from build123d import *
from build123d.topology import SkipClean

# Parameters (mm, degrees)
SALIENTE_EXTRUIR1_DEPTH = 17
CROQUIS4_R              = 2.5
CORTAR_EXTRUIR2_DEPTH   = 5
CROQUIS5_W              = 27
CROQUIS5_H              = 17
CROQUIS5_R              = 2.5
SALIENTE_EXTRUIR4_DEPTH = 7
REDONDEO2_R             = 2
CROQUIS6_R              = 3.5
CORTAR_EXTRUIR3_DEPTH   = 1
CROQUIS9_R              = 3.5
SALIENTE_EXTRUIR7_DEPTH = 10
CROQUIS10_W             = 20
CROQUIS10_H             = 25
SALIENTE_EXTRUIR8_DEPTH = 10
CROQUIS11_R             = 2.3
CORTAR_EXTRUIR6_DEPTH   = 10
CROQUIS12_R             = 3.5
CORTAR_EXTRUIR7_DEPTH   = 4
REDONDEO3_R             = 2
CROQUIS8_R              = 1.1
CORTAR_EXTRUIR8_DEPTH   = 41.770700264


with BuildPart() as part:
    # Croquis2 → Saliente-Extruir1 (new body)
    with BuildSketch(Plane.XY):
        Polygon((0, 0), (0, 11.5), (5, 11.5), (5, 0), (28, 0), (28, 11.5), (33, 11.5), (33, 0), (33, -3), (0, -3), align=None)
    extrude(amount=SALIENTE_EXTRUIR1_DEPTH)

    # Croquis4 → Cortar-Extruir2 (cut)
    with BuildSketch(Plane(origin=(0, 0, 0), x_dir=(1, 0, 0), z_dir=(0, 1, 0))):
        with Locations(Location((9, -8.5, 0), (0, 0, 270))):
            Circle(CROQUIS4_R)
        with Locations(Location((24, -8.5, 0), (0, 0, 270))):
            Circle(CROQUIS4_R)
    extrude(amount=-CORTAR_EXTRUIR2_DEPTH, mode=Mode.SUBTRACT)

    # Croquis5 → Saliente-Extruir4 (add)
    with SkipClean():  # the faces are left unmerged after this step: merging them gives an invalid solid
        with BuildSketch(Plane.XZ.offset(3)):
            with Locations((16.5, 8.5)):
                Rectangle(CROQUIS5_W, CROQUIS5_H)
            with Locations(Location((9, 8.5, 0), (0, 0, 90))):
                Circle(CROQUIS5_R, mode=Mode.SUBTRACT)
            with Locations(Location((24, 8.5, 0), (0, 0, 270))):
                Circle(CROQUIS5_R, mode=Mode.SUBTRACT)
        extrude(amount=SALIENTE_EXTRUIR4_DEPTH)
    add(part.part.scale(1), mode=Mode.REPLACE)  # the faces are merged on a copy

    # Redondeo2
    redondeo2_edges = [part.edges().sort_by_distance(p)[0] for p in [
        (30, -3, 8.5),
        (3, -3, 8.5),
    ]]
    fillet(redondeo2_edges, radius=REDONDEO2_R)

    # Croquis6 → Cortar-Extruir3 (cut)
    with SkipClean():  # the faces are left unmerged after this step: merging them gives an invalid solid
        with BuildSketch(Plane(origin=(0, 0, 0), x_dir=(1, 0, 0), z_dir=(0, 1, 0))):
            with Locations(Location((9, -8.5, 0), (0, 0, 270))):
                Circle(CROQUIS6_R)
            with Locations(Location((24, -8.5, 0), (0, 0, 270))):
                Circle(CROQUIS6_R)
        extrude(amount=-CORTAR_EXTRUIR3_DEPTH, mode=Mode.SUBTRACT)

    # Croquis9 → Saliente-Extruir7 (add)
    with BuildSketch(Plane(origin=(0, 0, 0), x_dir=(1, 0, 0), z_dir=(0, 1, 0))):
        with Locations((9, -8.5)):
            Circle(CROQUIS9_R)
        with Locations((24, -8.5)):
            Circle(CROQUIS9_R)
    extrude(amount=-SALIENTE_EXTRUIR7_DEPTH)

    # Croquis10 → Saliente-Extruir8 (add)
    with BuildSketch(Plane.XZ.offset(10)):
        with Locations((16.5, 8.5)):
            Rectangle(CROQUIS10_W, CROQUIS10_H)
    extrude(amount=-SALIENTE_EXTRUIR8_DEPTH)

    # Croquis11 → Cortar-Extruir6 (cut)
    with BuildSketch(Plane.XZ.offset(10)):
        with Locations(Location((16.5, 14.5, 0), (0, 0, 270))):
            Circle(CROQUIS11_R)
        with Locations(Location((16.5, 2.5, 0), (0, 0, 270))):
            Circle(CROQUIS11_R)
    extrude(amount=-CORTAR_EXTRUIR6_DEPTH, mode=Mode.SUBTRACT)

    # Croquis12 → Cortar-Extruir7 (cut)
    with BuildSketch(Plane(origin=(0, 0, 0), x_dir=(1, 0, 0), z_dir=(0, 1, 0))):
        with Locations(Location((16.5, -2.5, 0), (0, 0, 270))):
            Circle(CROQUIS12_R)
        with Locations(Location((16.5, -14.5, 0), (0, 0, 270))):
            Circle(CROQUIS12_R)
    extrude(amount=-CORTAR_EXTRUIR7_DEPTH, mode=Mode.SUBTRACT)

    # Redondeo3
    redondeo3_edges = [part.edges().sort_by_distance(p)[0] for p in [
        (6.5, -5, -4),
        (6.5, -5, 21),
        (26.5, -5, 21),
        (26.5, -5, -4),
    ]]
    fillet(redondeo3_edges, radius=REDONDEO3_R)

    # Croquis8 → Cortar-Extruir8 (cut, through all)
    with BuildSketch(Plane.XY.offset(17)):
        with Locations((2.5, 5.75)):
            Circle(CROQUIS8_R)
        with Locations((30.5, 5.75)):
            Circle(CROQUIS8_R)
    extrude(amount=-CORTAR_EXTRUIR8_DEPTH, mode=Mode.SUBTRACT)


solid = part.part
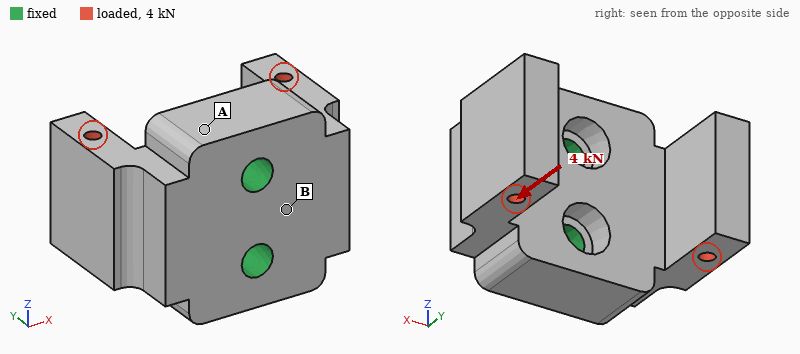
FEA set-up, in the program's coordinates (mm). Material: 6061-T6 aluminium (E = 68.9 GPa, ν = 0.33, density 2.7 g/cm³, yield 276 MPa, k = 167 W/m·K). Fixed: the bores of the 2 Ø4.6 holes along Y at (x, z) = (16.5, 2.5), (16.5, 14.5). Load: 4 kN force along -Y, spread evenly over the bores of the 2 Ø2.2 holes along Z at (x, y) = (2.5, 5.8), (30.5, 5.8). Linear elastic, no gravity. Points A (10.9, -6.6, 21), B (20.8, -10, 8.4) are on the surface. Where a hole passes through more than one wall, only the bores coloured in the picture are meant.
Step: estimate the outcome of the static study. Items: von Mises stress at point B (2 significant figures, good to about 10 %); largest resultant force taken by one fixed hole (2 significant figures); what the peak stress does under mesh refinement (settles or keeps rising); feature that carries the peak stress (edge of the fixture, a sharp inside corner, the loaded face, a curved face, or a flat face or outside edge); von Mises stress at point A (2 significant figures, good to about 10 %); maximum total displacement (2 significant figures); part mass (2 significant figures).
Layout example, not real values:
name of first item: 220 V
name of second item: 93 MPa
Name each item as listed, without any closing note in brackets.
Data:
von Mises stress at point B: 49 MPa
largest resultant force taken by one fixed hole: 2.0 kN
what the peak stress does under mesh refinement: keeps rising
feature that carries the peak stress: edge of the fixture
von Mises stress at point A: 20 MPa
maximum total displacement: 59 µm
part mass: 21 g
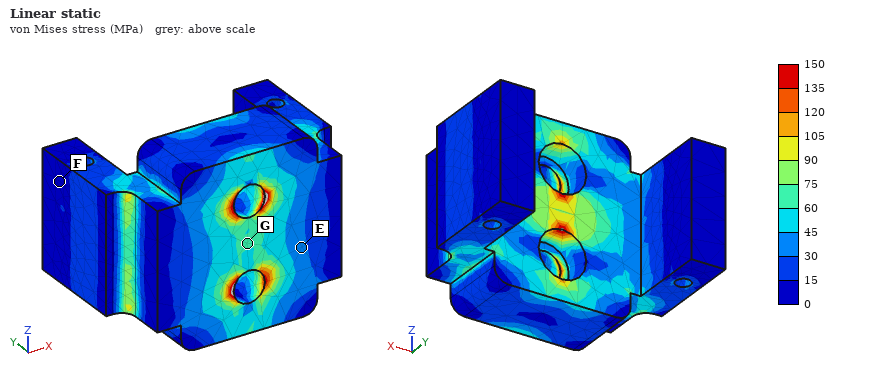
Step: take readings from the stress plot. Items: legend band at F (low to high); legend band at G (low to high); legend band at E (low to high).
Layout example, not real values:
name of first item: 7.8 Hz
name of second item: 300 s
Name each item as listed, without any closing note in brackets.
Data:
legend band at F: 0 to 15 MPa
legend band at G: 60 to 75 MPa
legend band at E: 30 to 45 MPa
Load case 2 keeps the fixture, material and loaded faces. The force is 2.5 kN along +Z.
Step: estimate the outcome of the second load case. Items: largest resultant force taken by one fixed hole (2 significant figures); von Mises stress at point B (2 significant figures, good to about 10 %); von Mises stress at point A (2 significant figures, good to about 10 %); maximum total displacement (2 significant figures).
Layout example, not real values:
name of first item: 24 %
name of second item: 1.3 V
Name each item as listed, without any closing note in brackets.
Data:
largest resultant force taken by one fixed hole: 2.3 kN
von Mises stress at point B: 13 MPa
von Mises stress at point A: 20 MPa
maximum total displacement: 41 µm
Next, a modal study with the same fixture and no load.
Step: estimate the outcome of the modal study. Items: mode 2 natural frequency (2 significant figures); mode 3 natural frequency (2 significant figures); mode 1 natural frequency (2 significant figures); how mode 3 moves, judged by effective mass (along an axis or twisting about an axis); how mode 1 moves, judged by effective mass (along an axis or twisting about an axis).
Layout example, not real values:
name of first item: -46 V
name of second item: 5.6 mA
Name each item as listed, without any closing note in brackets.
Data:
mode 2 natural frequency: 13 kHz
mode 3 natural frequency: 19 kHz
mode 1 natural frequency: 10 kHz
how mode 3 moves, judged by effective mass: along Z
how mode 1 moves, judged by effective mass: along X
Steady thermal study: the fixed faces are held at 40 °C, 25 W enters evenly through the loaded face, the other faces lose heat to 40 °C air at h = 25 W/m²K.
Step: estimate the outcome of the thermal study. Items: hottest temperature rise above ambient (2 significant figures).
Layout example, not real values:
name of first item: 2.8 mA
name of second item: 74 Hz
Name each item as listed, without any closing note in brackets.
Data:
hottest temperature rise above ambient: 14 K
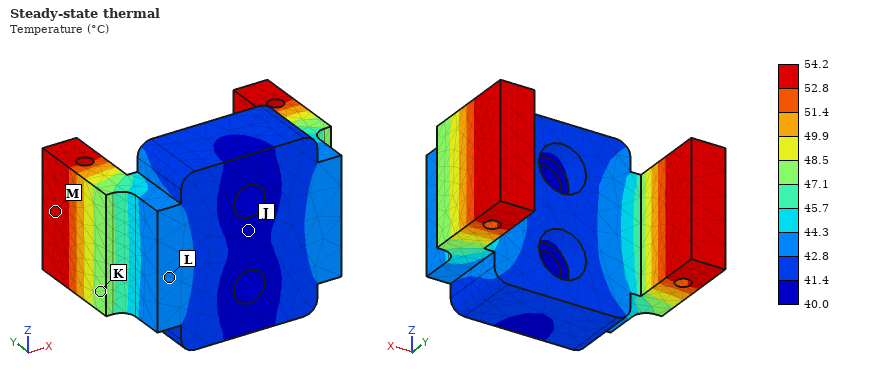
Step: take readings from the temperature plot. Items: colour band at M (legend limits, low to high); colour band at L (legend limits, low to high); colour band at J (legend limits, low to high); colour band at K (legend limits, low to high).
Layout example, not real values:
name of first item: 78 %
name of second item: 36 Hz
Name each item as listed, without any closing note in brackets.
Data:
colour band at M: 52.8 to 54.2 °C
colour band at L: 42.8 to 44.3 °C
colour band at J: 40.0 to 41.4 °C
colour band at K: 47.1 to 48.5 °C
